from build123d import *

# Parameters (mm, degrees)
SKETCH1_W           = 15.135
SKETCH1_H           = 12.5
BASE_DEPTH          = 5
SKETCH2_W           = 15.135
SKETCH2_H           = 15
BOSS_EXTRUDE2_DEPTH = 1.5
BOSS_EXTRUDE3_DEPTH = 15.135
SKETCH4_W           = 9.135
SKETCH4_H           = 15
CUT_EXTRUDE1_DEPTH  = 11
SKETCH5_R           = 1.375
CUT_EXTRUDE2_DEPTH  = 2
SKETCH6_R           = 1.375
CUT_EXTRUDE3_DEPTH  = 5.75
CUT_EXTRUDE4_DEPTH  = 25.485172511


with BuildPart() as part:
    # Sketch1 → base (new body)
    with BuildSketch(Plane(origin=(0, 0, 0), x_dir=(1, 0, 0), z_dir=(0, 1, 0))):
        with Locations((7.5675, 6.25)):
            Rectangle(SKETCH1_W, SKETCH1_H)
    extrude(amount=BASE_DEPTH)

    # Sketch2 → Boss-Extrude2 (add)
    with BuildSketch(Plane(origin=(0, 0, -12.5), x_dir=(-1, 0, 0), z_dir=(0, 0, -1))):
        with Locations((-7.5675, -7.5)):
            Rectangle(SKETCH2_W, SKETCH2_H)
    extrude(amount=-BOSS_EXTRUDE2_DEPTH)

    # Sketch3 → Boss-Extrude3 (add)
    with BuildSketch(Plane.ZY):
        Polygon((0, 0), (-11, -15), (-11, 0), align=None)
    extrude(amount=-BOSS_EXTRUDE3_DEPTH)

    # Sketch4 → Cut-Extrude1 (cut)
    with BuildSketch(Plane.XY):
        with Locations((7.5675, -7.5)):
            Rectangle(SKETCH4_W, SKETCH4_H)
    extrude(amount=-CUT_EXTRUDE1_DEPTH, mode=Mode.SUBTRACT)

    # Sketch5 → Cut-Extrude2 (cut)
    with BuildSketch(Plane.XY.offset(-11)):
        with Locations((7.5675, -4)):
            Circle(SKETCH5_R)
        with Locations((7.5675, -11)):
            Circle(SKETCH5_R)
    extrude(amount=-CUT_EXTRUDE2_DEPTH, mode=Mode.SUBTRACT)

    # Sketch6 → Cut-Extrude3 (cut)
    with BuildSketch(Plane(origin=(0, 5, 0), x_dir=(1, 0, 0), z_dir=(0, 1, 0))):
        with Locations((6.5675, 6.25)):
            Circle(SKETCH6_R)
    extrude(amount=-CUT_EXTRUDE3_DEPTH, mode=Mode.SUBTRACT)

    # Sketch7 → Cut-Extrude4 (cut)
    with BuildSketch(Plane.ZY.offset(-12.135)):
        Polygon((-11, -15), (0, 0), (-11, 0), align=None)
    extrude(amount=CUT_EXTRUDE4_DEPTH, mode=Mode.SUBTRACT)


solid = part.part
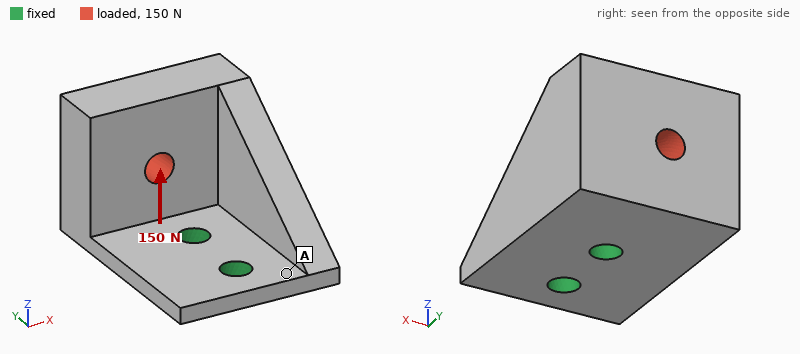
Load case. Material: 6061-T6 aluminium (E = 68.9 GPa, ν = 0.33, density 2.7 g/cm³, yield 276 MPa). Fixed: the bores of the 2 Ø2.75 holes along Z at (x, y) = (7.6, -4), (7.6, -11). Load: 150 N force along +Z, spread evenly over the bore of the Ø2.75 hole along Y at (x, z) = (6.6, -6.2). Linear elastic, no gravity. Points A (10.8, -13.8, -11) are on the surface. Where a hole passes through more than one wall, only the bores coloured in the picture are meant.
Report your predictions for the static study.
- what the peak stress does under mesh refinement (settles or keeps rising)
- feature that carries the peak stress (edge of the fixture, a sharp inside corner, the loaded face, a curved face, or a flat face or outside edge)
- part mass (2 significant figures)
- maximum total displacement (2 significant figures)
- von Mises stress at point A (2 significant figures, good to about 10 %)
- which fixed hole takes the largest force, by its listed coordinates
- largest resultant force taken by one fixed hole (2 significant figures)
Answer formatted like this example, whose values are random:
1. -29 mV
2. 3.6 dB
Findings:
1. keeps rising
2. edge of the fixture
3. 4.0 g
4. 33 µm
5. 14 MPa
6. (7.6, -4)
7. 220 N
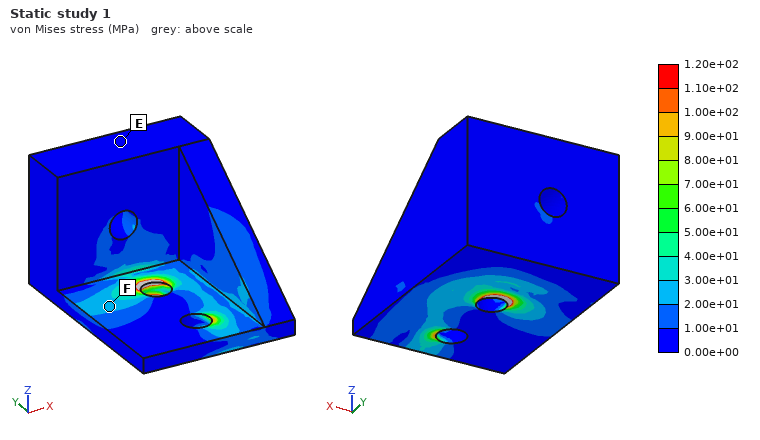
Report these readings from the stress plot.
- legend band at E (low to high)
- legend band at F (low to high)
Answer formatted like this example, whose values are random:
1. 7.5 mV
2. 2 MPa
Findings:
1. 0.00e+00 to 1.00e+01 MPa
2. 2.00e+01 to 3.00e+01 MPa
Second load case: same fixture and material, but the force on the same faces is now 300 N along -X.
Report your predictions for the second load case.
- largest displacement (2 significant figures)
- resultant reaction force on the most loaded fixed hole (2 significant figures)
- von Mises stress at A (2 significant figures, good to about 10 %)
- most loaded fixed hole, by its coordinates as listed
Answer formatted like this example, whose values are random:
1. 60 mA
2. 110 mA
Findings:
1. 0.12 mm
2. 460 N
3. 64 MPa
4. (7.6, -4)
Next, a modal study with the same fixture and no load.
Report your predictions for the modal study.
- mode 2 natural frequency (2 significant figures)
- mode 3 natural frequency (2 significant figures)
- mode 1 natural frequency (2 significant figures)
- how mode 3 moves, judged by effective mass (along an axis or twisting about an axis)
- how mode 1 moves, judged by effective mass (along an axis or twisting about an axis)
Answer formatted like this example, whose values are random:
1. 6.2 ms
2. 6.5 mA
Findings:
1. 7300 Hz
2. 18 kHz
3. 5100 Hz
4. along Z
5. along X
